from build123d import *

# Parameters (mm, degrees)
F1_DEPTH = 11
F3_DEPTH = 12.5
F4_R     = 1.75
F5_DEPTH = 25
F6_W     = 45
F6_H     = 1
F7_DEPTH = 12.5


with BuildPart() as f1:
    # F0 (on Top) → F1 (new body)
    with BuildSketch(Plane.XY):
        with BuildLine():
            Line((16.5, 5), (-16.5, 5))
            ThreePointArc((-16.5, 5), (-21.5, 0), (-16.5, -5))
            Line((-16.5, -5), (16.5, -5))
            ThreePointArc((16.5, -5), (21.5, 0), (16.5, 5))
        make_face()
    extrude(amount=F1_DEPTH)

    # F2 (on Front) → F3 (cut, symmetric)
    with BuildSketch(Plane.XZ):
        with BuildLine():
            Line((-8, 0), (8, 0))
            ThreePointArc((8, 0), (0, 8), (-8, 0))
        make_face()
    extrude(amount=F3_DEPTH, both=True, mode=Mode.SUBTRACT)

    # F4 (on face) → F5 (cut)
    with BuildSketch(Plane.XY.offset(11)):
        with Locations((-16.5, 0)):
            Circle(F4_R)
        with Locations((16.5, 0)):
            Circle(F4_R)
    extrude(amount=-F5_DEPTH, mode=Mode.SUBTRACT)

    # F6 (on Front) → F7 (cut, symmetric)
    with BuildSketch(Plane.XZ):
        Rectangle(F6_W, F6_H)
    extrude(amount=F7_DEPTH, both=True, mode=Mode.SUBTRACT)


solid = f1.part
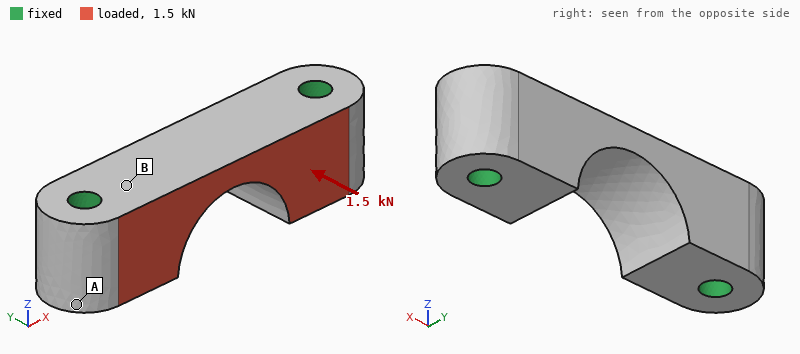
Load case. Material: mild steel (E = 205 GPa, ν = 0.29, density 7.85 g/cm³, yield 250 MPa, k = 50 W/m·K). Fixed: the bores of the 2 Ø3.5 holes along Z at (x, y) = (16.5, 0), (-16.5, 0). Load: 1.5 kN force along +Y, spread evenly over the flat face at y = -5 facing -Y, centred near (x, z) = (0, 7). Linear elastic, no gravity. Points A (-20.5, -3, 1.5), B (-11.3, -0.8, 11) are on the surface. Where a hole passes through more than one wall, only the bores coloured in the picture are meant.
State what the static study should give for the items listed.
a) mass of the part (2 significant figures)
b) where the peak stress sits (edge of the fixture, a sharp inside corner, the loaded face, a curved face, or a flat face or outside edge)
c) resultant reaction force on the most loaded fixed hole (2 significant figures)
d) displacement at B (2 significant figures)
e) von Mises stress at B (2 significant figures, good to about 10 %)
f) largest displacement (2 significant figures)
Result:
25 g
edge of the fixture
750 N
0.96 µm
16 MPa
2.7 µm
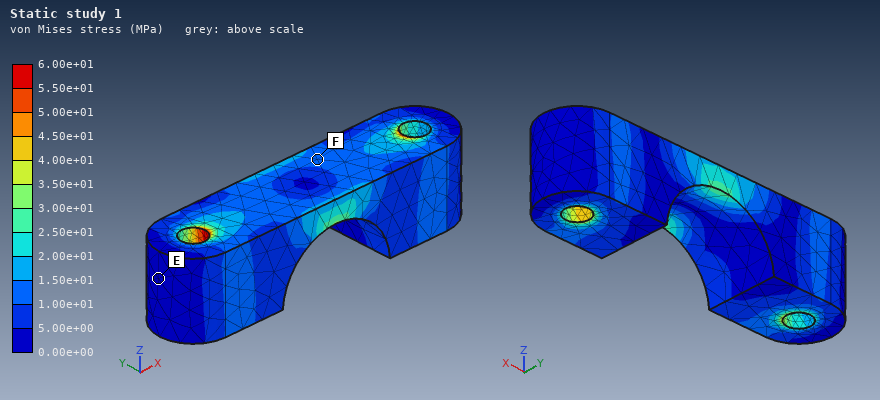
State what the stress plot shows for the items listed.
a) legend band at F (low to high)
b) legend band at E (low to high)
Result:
1.00e+01 to 1.50e+01 MPa
0.00e+00 to 5.00e+00 MPa
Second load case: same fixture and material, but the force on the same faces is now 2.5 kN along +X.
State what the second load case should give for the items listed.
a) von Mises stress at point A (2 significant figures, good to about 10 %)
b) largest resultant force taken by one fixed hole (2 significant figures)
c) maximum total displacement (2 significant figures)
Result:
5.9 MPa
1.3 kN
1.5 µm
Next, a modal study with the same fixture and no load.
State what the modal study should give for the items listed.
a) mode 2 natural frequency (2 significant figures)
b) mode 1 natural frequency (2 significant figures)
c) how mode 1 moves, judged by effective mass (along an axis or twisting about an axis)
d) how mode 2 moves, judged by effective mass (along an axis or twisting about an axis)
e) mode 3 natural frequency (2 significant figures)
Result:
43 kHz
33 kHz
along Y
along Z
59 kHz
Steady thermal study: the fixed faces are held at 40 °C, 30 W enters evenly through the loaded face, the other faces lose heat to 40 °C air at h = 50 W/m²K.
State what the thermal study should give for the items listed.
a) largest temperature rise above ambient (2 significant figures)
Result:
29 K
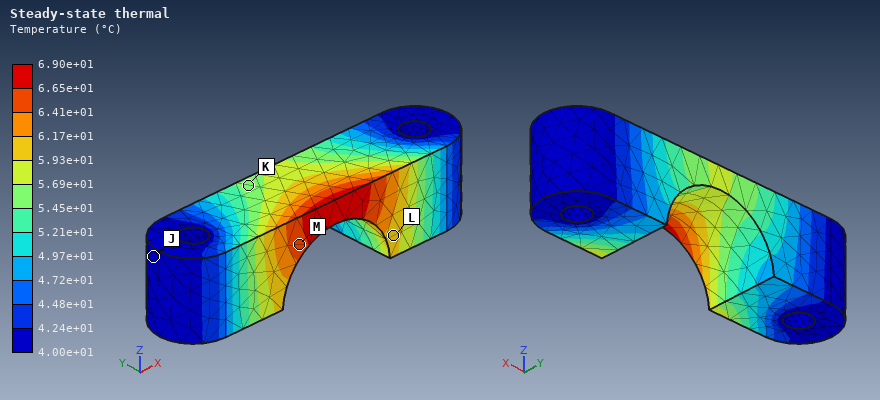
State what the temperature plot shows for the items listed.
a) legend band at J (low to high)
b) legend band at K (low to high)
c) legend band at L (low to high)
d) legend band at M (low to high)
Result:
4.00e+01 to 4.24e+01 °C
5.45e+01 to 5.69e+01 °C
5.93e+01 to 6.17e+01 °C
6.41e+01 to 6.65e+01 °C
